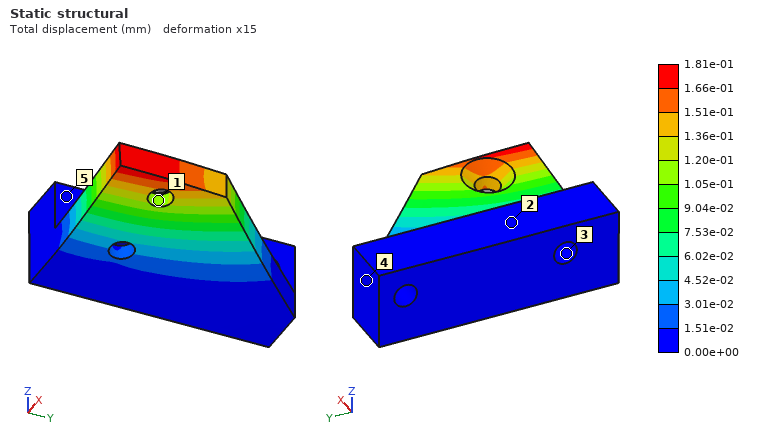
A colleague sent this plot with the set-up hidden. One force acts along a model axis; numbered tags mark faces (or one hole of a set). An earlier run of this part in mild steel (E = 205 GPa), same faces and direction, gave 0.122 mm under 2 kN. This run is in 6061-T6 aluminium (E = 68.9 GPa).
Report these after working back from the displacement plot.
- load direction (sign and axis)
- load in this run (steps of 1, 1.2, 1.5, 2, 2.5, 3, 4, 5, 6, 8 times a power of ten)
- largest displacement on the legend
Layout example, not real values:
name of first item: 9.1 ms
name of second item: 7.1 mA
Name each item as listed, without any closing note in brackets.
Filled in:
load direction: +Z
load in this run: 1 kN
largest displacement on the legend: 1.81e-01 mm
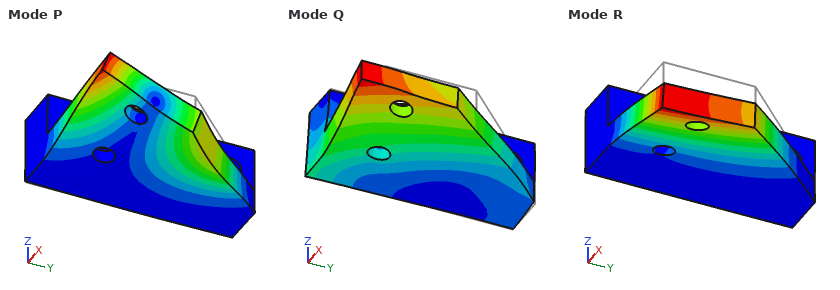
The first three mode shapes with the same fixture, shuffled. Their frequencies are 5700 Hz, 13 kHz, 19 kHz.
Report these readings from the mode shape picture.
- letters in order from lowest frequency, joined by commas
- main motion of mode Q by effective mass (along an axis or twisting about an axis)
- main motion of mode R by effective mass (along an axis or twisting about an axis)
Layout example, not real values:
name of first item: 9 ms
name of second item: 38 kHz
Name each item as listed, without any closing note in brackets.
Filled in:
letters in order from lowest frequency, joined by commas: R, P, Q
main motion of mode Q by effective mass: along Y
main motion of mode R by effective mass: along Z
